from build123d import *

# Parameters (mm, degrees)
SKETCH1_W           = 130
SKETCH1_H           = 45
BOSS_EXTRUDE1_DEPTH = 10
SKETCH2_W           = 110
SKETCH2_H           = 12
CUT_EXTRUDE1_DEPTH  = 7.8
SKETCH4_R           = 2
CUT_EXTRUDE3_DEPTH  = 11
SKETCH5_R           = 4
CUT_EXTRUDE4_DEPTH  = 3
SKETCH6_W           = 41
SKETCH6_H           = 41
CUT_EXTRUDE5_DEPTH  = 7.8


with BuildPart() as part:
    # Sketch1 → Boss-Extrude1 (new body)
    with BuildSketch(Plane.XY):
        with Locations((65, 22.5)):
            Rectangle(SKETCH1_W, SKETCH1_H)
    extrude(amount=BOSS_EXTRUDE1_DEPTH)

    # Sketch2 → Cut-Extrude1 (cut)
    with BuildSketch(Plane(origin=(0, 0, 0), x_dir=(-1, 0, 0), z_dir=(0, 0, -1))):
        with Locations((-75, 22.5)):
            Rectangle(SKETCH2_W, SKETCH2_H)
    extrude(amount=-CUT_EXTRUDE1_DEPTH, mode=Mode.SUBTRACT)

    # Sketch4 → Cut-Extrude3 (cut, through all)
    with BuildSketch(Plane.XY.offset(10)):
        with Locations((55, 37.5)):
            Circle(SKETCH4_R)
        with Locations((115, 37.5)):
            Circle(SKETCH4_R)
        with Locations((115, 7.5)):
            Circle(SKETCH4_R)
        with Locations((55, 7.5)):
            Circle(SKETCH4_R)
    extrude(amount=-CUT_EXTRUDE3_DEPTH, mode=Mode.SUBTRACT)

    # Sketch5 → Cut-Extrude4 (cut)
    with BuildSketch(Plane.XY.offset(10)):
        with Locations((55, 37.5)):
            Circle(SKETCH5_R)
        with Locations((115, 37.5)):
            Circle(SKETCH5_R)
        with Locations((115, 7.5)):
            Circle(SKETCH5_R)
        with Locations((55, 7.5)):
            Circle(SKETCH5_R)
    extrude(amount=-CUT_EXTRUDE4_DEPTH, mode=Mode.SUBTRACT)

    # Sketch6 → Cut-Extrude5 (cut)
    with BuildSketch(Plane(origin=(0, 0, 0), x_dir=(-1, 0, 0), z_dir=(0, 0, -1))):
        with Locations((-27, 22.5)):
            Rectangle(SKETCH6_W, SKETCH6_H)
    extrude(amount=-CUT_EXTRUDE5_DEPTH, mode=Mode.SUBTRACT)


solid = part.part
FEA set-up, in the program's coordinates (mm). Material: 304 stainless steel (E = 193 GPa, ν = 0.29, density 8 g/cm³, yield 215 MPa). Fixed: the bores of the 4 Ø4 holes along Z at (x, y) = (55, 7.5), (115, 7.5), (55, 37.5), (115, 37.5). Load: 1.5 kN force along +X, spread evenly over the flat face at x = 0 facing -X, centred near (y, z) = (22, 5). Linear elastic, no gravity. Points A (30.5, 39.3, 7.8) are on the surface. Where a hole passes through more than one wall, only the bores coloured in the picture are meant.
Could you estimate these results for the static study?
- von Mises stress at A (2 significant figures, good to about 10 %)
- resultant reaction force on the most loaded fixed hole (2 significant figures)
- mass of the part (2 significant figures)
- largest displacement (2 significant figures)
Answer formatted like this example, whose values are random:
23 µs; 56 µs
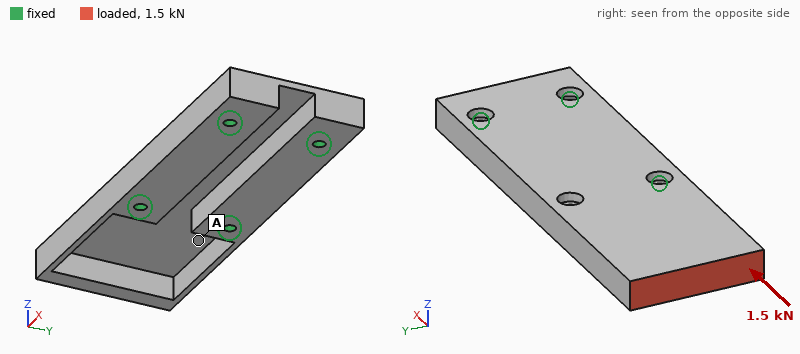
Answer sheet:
11 MPa; 670 N; 290 g; 45 µm
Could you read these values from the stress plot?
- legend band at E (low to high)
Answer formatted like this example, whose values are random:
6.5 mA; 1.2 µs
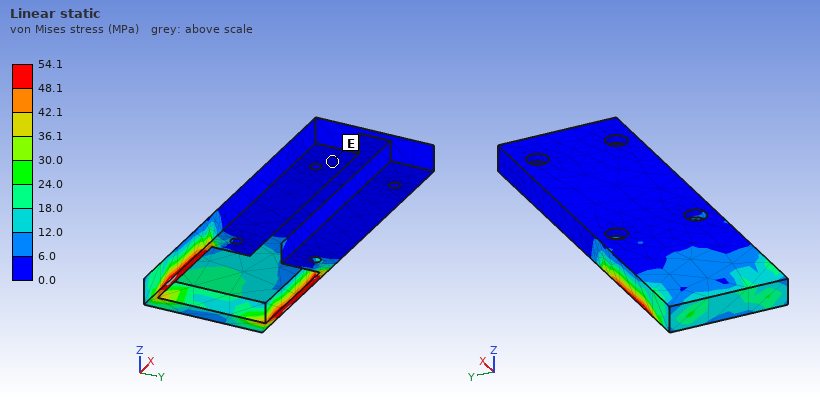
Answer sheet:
0.0 to 6.0 MPa
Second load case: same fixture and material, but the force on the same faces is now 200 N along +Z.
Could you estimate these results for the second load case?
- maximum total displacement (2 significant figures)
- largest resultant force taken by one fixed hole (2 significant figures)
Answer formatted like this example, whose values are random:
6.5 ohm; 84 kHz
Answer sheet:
81 µm; 180 N
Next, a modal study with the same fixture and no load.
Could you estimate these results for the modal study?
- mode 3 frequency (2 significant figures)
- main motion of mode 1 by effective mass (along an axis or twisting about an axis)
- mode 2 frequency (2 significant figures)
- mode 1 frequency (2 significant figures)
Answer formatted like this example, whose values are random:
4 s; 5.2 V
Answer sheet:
6600 Hz; along Z; 2700 Hz; 1500 Hz
